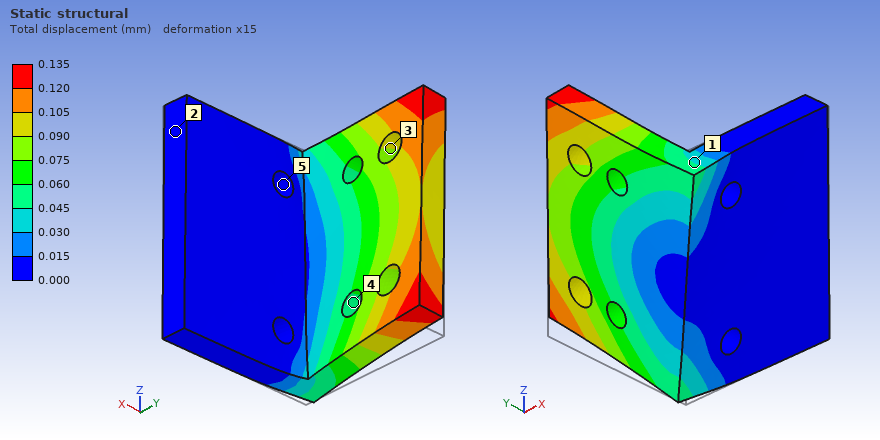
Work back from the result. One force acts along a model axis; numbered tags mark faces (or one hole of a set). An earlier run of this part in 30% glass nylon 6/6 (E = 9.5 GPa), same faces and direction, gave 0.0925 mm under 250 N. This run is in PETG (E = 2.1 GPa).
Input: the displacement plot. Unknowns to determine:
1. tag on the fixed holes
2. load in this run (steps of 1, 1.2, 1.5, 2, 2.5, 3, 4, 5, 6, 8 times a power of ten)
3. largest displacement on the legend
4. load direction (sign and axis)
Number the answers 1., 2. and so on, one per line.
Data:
1. 5
2. 80 N
3. 0.135 mm
4. +Z
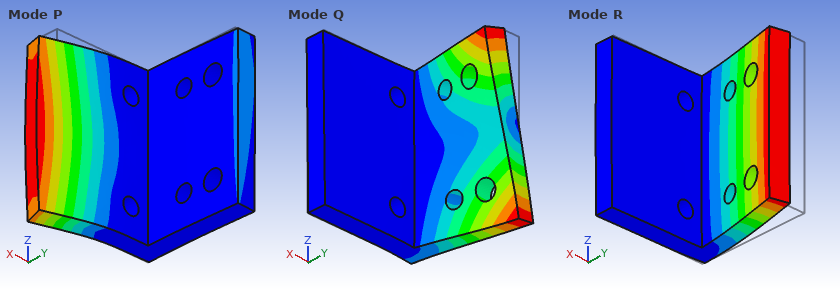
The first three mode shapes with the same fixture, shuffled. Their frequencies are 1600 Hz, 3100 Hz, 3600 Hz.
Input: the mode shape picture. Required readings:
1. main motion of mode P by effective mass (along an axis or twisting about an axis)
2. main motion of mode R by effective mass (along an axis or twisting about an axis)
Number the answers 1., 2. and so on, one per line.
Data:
1. along Y
2. along X
